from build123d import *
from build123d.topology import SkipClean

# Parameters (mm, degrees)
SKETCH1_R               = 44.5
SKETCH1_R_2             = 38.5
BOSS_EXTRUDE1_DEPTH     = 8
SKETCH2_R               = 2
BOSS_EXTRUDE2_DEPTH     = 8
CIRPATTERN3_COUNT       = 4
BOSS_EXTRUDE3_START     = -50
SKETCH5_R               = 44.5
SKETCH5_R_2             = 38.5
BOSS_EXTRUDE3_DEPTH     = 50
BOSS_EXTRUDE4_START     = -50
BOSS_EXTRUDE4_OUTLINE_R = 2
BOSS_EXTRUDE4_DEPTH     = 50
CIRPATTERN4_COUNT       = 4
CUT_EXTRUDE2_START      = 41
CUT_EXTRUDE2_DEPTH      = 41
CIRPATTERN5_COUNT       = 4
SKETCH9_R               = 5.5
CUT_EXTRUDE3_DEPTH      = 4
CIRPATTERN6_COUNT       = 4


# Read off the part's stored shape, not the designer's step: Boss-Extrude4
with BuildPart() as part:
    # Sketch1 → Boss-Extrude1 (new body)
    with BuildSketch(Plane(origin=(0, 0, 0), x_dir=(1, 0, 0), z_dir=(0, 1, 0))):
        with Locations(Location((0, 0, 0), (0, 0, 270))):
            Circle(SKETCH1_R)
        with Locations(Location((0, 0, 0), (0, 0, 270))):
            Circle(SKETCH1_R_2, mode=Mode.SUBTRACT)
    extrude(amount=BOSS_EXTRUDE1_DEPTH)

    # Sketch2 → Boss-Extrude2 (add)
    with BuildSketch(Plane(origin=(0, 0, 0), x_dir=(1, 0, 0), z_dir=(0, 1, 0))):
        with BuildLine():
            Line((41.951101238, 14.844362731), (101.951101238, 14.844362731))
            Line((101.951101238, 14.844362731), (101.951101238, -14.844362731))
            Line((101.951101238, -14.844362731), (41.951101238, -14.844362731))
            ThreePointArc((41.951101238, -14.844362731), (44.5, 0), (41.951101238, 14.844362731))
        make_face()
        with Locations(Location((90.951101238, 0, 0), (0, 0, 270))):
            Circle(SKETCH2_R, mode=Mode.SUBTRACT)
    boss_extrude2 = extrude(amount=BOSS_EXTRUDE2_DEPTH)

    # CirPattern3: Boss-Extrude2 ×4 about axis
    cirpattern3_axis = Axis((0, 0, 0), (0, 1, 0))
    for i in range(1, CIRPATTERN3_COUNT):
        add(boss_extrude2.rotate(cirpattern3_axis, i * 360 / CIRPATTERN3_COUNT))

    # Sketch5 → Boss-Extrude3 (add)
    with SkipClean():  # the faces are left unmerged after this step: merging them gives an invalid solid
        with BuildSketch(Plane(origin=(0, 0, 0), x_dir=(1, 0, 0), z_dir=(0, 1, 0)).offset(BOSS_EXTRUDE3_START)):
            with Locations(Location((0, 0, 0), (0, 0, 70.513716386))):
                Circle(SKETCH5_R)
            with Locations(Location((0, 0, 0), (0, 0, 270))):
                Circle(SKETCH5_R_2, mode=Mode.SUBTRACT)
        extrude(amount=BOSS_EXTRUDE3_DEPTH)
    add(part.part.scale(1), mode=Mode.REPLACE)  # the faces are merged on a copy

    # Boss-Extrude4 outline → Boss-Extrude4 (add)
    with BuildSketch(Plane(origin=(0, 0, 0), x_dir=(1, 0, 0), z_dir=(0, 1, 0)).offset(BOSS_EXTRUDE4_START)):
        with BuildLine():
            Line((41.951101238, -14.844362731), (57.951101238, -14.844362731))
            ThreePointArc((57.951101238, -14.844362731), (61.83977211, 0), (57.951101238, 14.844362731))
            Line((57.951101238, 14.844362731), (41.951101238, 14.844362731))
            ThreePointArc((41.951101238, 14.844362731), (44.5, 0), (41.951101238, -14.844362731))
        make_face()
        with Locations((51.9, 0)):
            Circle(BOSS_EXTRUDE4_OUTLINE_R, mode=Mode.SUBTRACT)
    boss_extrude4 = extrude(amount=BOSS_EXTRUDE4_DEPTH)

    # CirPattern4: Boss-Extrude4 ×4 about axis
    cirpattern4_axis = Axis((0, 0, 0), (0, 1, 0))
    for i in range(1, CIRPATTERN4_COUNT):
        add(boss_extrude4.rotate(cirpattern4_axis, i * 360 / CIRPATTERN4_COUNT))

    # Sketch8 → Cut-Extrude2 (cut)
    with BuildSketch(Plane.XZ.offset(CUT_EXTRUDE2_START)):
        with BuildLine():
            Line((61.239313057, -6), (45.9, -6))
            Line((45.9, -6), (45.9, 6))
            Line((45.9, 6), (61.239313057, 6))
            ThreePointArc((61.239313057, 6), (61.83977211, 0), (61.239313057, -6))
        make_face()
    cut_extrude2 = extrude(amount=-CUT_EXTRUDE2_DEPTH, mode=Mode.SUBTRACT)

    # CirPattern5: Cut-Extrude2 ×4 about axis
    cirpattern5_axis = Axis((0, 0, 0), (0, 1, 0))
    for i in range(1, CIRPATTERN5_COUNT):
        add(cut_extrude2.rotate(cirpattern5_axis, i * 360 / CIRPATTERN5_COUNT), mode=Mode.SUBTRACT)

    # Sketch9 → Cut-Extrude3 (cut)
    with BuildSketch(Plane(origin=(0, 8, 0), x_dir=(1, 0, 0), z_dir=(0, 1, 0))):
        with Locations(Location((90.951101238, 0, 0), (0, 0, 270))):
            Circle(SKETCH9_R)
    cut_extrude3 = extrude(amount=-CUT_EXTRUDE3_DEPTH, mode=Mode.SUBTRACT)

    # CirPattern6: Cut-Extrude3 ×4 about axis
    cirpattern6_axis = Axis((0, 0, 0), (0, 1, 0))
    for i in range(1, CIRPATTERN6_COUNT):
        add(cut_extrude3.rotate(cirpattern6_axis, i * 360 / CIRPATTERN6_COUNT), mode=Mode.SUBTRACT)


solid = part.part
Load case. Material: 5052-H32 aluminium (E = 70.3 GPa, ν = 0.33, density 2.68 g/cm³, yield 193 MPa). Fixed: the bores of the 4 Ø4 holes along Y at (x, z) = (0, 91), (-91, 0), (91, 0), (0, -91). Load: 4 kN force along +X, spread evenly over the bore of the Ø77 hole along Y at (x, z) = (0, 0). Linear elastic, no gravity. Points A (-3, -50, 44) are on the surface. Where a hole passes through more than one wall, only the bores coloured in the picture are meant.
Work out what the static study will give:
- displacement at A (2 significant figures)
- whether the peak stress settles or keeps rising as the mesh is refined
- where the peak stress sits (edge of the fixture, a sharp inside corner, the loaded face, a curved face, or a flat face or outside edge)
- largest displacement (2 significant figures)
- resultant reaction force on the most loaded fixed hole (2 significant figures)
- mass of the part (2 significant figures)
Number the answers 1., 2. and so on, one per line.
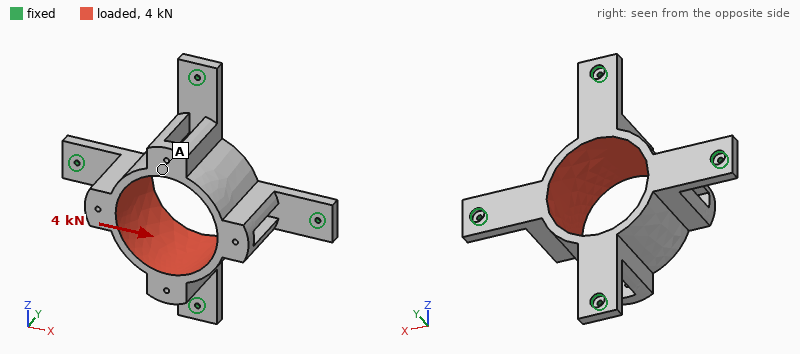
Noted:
1. 63 µm
2. keeps rising
3. edge of the fixture
4. 78 µm
5. 2.0 kN
6. 570 g
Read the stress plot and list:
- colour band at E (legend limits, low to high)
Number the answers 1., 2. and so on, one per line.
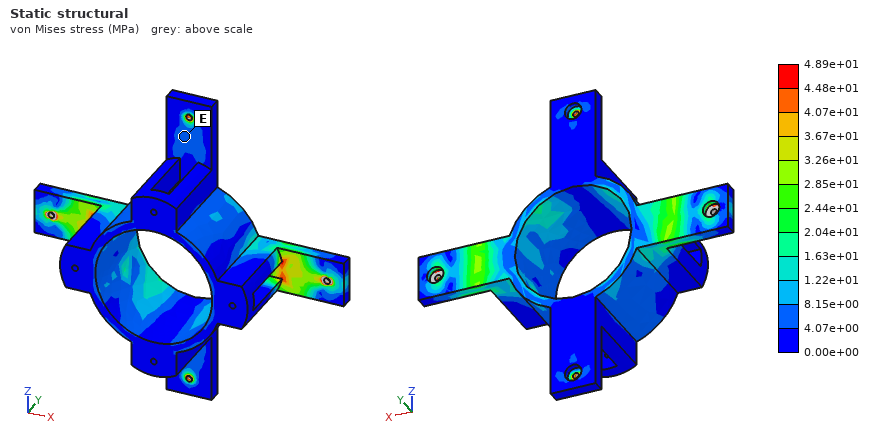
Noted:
1. 4.07e+00 to 8.15e+00 MPa
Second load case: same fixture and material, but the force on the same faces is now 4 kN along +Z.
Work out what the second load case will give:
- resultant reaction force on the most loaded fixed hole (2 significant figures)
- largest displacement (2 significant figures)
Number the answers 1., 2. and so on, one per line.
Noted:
1. 2.0 kN
2. 78 µm
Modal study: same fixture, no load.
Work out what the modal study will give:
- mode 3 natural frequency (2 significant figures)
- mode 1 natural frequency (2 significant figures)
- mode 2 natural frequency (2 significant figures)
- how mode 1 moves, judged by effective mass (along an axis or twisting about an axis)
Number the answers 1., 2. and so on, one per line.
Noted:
1. 1700 Hz
2. 1300 Hz
3. 1700 Hz
4. along Y
